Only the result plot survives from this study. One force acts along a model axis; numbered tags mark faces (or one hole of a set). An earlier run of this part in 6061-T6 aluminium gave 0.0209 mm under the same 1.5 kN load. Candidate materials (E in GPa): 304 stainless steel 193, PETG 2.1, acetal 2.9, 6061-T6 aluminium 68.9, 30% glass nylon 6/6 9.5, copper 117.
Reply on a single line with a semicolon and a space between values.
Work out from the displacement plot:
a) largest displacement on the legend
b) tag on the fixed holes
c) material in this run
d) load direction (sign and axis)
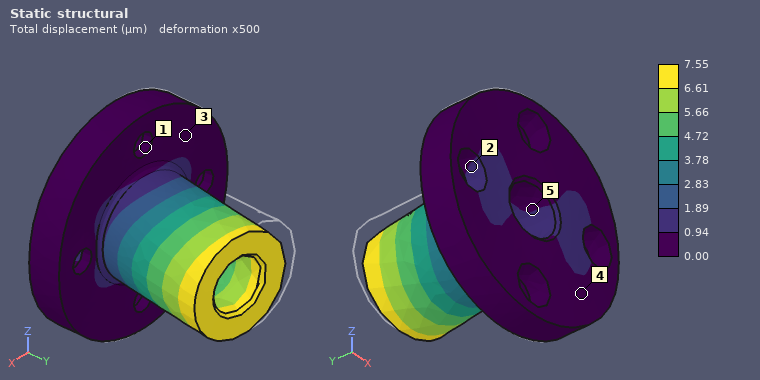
7.55 µm; 1; 304 stainless steel; +X
